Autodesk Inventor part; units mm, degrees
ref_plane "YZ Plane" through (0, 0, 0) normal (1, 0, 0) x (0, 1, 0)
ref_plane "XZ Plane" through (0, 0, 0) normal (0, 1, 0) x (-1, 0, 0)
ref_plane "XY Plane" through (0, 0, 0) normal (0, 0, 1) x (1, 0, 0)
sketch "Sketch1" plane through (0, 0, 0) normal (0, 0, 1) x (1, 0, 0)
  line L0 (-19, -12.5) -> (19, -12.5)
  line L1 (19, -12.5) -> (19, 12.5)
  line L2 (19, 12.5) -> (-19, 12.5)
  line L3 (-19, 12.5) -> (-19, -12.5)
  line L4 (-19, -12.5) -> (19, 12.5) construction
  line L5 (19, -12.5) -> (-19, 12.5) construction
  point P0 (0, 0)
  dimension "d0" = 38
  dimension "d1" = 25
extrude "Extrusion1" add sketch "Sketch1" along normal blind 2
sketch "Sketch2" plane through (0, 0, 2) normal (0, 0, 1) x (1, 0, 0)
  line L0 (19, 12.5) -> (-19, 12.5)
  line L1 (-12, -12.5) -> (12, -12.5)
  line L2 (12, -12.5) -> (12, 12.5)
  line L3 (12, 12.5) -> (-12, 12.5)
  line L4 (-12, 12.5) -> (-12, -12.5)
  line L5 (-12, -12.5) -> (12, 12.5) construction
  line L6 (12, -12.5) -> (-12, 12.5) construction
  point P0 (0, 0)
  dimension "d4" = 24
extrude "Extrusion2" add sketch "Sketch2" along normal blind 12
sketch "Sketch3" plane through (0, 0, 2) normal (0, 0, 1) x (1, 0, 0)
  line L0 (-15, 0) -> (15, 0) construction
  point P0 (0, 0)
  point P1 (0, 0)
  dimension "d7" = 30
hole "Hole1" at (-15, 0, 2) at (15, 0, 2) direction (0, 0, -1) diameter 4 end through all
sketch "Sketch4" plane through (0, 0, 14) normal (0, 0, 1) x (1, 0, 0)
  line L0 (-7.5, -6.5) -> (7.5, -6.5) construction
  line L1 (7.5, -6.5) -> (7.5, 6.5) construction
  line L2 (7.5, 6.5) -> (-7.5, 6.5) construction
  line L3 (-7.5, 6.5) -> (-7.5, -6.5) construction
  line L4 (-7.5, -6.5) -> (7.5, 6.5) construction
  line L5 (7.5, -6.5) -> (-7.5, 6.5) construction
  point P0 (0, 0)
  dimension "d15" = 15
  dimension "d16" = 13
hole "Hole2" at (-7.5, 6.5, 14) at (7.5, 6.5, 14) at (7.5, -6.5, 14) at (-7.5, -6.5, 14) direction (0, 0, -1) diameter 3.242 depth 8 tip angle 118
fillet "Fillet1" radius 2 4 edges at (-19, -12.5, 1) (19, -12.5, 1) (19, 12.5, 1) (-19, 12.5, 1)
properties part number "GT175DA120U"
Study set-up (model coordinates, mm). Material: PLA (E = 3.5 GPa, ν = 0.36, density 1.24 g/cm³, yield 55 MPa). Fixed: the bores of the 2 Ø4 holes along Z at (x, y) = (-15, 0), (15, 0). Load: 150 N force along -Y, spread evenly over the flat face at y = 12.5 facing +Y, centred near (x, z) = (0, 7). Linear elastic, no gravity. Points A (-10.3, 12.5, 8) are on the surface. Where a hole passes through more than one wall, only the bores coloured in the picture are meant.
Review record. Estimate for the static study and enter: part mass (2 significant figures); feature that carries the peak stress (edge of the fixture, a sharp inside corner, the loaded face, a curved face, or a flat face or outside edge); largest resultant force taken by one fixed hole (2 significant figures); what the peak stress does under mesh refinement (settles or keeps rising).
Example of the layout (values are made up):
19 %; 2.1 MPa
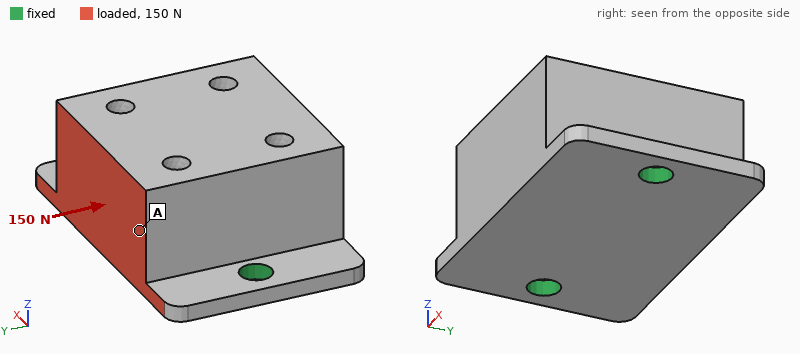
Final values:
11 g; edge of the fixture; 75 N; keeps rising
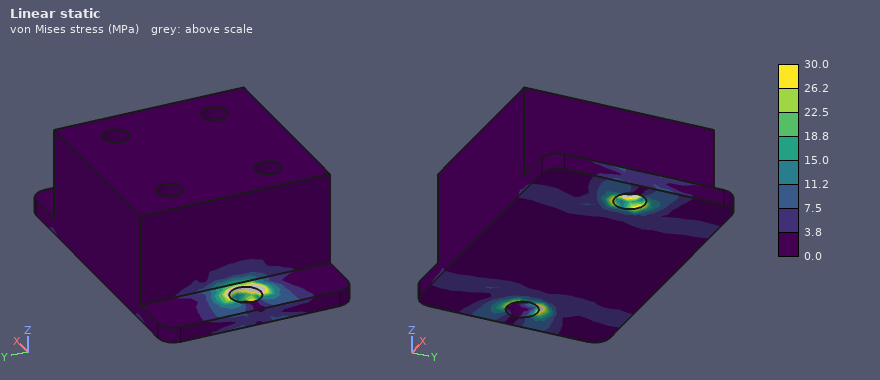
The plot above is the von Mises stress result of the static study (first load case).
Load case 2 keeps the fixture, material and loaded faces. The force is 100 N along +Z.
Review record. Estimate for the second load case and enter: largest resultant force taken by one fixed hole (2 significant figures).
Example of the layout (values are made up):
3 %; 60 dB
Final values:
58 N
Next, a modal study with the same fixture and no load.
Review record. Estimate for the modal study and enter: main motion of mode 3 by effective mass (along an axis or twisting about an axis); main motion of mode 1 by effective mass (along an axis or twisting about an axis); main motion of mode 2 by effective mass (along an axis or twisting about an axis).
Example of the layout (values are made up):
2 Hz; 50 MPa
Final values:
along X; along Y; along Z
